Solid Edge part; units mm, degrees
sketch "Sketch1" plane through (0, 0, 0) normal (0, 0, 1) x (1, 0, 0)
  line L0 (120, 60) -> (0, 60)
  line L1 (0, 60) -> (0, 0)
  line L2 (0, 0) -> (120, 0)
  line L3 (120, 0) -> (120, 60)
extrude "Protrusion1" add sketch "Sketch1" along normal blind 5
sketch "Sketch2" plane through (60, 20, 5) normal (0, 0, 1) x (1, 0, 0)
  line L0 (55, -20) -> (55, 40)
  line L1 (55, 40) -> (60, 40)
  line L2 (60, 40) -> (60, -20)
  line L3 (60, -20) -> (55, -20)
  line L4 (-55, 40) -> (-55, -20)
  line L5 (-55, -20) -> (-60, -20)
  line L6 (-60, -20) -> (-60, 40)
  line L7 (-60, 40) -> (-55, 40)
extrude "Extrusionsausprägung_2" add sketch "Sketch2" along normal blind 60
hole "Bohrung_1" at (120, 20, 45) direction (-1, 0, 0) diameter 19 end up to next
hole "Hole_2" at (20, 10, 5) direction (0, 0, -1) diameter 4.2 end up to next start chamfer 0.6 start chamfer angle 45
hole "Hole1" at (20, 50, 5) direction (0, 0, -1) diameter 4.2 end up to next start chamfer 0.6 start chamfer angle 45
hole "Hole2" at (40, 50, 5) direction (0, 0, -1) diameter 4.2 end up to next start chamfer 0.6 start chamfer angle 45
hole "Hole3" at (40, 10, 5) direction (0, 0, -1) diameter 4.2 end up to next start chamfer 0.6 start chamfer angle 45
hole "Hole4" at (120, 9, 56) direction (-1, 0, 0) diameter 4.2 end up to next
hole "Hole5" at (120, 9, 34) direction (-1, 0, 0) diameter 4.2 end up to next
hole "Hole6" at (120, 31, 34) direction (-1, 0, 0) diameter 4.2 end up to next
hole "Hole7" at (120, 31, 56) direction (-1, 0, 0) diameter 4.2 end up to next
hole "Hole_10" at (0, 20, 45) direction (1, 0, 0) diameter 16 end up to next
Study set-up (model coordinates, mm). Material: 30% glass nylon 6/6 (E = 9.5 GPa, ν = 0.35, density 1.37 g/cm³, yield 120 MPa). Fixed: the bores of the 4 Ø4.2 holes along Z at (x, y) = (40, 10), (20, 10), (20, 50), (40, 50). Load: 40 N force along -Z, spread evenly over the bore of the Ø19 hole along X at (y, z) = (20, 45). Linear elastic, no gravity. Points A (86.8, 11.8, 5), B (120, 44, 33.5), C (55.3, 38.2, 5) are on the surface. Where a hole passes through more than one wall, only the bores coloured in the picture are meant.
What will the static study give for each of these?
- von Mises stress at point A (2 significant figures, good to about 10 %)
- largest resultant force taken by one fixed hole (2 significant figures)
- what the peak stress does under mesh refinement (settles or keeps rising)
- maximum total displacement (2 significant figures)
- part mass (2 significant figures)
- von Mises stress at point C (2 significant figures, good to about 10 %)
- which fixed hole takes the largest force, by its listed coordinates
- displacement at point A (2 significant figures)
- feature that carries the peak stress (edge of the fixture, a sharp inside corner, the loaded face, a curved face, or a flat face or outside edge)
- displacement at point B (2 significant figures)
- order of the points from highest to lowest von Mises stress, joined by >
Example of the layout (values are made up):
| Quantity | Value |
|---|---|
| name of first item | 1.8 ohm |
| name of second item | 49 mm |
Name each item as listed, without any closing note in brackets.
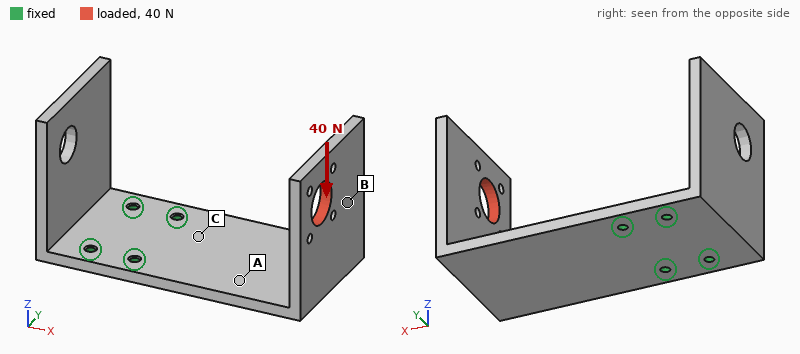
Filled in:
| Quantity | Value |
|---|---|
| von Mises stress at point A | 5.2 MPa |
| largest resultant force taken by one fixed hole | 64 N |
| what the peak stress does under mesh refinement | keeps rising |
| maximum total displacement | 1.8 mm |
| part mass | 95 g |
| von Mises stress at point C | 8.7 MPa |
| which fixed hole takes the largest force, by its listed coordinates | (40, 10) |
| displacement at point A | 0.51 mm |
| feature that carries the peak stress | edge of the fixture |
| displacement at point B | 1.3 mm |
| order of the points from highest to lowest von Mises stress, joined by > | C > A > B |
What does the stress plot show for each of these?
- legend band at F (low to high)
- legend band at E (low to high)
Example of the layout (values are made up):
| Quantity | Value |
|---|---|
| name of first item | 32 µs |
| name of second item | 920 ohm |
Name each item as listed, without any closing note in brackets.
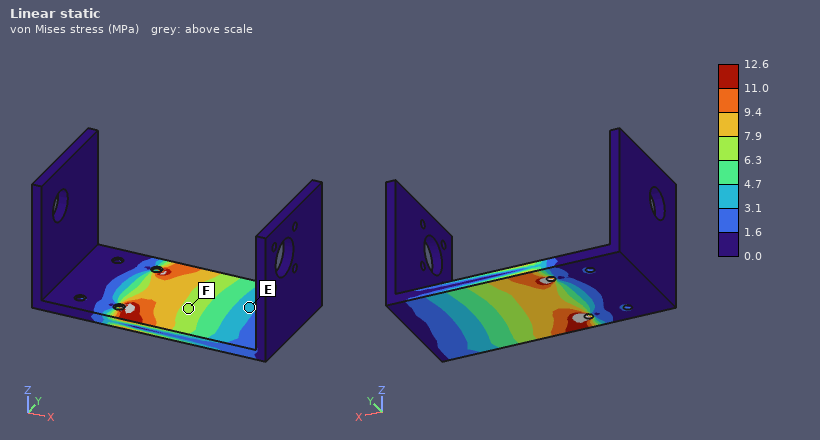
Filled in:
| Quantity | Value |
|---|---|
| legend band at F | 6.3 to 7.9 MPa |
| legend band at E | 3.1 to 4.7 MPa |
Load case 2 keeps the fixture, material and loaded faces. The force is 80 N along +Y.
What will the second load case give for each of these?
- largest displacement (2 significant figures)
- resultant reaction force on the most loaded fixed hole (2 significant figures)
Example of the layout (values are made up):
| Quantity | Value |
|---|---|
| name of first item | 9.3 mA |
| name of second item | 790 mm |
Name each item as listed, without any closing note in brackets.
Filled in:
| Quantity | Value |
|---|---|
| largest displacement | 1.6 mm |
| resultant reaction force on the most loaded fixed hole | 160 N |
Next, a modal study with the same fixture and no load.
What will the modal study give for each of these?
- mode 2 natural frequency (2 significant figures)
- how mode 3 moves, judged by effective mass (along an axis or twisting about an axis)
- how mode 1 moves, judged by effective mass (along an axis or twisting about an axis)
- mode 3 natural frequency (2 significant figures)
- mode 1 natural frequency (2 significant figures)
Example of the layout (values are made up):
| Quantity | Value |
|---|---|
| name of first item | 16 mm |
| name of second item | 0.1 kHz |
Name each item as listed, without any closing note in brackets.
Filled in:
| Quantity | Value |
|---|---|
| mode 2 natural frequency | 310 Hz |
| how mode 3 moves, judged by effective mass | along X |
| how mode 1 moves, judged by effective mass | along Z |
| mode 3 natural frequency | 400 Hz |
| mode 1 natural frequency | 150 Hz |
